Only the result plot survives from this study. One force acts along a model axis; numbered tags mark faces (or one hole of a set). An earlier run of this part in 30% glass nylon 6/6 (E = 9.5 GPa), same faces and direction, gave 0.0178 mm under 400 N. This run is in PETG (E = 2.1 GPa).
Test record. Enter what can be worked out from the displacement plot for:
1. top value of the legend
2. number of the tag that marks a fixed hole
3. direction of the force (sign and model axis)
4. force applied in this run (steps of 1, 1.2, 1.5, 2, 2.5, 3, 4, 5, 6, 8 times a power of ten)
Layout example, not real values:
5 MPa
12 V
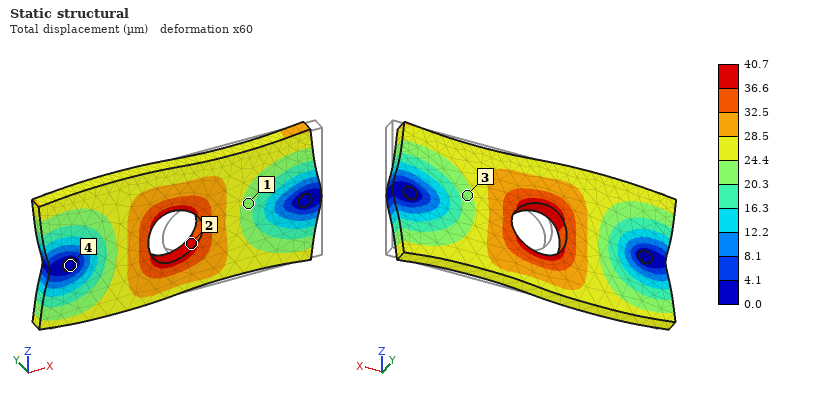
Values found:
40.7 µm
4
-X
200 N
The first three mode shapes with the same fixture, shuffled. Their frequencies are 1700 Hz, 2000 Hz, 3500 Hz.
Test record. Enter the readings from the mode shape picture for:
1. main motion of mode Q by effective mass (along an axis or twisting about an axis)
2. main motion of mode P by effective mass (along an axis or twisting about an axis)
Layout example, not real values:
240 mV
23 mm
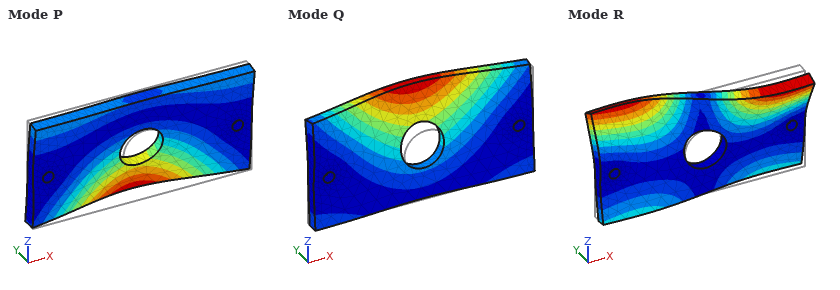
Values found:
along Y
along Y
